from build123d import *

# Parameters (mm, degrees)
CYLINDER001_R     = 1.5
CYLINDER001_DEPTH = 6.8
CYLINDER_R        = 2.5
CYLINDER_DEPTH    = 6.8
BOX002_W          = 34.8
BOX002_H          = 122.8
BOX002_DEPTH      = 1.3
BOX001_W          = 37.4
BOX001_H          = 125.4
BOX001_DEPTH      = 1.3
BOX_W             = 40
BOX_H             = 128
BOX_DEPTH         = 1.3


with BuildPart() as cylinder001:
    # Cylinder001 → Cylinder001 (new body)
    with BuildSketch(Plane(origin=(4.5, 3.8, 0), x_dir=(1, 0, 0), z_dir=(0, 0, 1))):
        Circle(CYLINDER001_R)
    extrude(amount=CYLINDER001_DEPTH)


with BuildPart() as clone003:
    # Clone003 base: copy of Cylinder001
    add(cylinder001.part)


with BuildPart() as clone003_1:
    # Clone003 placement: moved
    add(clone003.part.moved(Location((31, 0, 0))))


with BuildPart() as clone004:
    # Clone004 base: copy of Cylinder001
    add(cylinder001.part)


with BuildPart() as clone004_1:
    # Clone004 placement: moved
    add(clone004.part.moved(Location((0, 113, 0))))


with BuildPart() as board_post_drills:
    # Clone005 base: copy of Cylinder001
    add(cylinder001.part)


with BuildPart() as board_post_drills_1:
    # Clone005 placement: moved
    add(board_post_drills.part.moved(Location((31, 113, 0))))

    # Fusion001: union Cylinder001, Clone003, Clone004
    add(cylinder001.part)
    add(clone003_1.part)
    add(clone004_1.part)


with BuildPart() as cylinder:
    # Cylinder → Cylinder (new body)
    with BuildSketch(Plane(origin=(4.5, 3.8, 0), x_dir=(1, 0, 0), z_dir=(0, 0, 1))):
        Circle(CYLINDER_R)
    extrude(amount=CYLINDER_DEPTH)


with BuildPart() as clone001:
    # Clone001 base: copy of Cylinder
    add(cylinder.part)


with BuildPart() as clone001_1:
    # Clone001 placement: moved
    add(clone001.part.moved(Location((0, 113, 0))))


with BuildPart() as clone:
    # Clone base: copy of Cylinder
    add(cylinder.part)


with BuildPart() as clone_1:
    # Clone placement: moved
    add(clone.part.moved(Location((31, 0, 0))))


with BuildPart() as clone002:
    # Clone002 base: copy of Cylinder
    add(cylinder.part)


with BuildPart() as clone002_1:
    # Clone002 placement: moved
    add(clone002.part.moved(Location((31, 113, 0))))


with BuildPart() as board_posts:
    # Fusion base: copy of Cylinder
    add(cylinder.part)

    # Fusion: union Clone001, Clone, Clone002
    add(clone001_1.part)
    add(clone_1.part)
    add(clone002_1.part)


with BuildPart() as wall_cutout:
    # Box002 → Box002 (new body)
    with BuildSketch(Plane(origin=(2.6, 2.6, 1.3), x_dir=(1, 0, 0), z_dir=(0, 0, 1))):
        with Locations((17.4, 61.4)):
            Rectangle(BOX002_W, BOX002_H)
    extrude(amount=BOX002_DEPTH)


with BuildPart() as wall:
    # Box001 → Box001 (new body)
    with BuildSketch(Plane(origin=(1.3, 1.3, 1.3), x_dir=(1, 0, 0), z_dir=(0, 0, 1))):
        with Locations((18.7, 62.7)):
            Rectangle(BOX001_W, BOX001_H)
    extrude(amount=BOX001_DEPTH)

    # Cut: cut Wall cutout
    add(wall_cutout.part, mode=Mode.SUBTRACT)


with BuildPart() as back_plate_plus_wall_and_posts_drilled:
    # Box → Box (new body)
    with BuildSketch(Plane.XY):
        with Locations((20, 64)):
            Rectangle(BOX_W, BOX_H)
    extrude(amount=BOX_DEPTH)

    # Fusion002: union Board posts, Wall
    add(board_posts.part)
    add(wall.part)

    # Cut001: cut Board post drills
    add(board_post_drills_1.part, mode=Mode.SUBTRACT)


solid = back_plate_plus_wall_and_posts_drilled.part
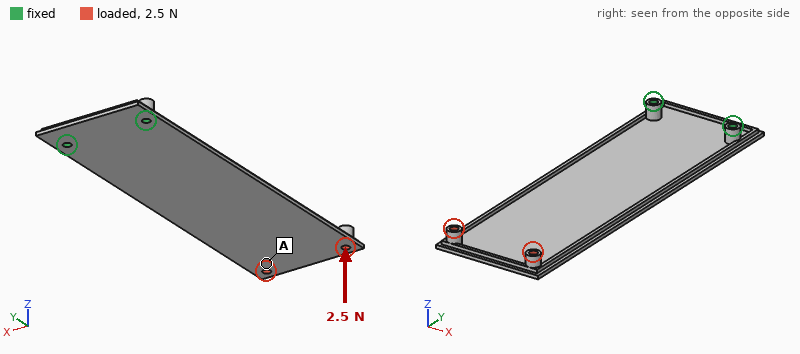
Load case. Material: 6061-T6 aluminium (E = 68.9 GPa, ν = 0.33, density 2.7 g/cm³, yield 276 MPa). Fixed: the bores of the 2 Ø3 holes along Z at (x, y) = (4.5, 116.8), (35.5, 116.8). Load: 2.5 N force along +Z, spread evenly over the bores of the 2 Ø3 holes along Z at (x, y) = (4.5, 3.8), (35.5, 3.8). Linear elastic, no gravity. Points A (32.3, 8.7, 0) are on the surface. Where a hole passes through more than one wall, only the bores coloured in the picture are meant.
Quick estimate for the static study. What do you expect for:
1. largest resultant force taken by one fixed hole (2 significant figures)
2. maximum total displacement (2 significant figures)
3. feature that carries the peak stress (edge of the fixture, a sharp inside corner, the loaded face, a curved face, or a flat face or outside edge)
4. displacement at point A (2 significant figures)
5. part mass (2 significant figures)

3.4 N
1.4 mm
a flat face or outside edge
1.2 mm
20 g
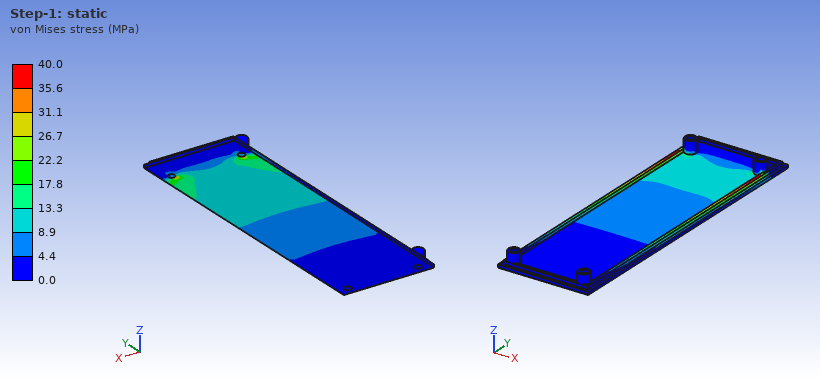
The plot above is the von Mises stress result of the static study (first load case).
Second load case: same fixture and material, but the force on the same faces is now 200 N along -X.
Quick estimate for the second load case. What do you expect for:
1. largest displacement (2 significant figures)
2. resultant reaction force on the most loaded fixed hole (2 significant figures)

1.4 mm
720 N
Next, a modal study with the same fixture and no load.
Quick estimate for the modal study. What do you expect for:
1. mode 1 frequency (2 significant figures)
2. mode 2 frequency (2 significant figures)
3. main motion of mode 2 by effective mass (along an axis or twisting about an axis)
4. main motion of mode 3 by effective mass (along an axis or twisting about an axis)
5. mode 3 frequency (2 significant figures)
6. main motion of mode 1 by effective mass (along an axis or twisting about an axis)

97 Hz
470 Hz
twisting about Y
along Z
620 Hz
along Z
